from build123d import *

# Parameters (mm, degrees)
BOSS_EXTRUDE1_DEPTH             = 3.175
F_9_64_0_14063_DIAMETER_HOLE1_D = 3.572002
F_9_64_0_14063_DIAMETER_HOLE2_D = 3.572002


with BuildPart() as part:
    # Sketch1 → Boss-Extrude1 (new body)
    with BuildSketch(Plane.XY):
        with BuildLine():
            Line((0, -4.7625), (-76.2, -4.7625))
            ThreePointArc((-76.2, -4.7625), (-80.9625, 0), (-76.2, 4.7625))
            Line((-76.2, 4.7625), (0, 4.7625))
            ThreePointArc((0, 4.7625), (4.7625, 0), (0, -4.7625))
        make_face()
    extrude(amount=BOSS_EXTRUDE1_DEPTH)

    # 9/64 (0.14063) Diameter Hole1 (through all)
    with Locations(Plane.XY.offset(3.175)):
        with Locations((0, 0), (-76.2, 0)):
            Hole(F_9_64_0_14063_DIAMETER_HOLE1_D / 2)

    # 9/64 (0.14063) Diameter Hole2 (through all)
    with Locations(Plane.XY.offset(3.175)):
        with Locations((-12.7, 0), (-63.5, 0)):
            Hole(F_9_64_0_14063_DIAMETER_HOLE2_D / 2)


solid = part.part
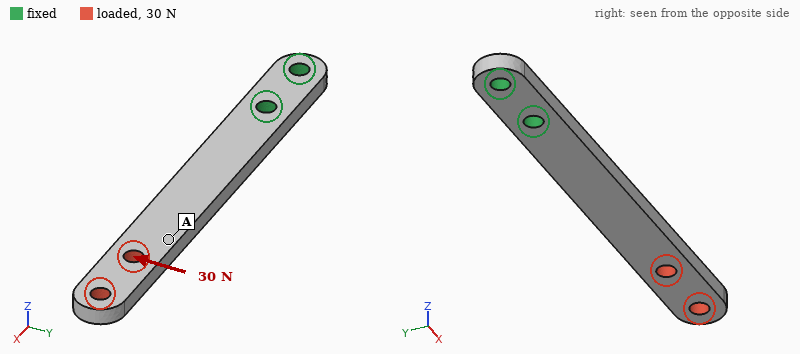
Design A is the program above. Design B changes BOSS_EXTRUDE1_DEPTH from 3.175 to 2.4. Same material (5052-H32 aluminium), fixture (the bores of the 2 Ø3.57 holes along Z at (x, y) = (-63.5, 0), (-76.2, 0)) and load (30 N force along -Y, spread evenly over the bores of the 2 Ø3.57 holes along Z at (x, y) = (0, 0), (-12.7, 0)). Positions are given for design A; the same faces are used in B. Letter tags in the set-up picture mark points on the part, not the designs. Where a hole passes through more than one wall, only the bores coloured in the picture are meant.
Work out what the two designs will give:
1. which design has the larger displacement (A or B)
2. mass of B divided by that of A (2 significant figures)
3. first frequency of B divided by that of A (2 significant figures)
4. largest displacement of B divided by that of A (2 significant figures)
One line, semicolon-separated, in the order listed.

B; 0.76; 0.76; 1.3
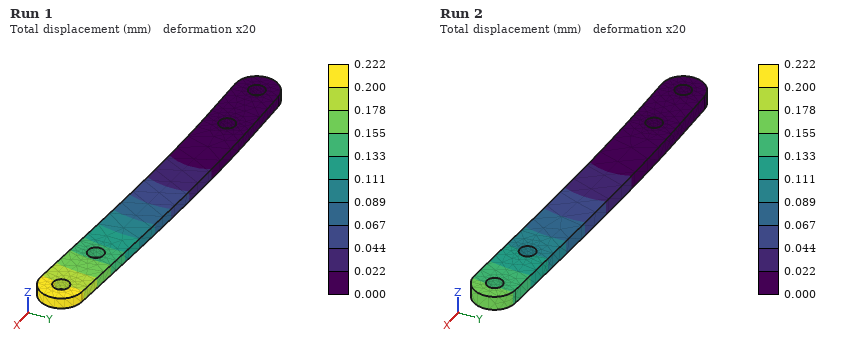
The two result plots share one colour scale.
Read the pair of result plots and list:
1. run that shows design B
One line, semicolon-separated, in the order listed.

Run 1
